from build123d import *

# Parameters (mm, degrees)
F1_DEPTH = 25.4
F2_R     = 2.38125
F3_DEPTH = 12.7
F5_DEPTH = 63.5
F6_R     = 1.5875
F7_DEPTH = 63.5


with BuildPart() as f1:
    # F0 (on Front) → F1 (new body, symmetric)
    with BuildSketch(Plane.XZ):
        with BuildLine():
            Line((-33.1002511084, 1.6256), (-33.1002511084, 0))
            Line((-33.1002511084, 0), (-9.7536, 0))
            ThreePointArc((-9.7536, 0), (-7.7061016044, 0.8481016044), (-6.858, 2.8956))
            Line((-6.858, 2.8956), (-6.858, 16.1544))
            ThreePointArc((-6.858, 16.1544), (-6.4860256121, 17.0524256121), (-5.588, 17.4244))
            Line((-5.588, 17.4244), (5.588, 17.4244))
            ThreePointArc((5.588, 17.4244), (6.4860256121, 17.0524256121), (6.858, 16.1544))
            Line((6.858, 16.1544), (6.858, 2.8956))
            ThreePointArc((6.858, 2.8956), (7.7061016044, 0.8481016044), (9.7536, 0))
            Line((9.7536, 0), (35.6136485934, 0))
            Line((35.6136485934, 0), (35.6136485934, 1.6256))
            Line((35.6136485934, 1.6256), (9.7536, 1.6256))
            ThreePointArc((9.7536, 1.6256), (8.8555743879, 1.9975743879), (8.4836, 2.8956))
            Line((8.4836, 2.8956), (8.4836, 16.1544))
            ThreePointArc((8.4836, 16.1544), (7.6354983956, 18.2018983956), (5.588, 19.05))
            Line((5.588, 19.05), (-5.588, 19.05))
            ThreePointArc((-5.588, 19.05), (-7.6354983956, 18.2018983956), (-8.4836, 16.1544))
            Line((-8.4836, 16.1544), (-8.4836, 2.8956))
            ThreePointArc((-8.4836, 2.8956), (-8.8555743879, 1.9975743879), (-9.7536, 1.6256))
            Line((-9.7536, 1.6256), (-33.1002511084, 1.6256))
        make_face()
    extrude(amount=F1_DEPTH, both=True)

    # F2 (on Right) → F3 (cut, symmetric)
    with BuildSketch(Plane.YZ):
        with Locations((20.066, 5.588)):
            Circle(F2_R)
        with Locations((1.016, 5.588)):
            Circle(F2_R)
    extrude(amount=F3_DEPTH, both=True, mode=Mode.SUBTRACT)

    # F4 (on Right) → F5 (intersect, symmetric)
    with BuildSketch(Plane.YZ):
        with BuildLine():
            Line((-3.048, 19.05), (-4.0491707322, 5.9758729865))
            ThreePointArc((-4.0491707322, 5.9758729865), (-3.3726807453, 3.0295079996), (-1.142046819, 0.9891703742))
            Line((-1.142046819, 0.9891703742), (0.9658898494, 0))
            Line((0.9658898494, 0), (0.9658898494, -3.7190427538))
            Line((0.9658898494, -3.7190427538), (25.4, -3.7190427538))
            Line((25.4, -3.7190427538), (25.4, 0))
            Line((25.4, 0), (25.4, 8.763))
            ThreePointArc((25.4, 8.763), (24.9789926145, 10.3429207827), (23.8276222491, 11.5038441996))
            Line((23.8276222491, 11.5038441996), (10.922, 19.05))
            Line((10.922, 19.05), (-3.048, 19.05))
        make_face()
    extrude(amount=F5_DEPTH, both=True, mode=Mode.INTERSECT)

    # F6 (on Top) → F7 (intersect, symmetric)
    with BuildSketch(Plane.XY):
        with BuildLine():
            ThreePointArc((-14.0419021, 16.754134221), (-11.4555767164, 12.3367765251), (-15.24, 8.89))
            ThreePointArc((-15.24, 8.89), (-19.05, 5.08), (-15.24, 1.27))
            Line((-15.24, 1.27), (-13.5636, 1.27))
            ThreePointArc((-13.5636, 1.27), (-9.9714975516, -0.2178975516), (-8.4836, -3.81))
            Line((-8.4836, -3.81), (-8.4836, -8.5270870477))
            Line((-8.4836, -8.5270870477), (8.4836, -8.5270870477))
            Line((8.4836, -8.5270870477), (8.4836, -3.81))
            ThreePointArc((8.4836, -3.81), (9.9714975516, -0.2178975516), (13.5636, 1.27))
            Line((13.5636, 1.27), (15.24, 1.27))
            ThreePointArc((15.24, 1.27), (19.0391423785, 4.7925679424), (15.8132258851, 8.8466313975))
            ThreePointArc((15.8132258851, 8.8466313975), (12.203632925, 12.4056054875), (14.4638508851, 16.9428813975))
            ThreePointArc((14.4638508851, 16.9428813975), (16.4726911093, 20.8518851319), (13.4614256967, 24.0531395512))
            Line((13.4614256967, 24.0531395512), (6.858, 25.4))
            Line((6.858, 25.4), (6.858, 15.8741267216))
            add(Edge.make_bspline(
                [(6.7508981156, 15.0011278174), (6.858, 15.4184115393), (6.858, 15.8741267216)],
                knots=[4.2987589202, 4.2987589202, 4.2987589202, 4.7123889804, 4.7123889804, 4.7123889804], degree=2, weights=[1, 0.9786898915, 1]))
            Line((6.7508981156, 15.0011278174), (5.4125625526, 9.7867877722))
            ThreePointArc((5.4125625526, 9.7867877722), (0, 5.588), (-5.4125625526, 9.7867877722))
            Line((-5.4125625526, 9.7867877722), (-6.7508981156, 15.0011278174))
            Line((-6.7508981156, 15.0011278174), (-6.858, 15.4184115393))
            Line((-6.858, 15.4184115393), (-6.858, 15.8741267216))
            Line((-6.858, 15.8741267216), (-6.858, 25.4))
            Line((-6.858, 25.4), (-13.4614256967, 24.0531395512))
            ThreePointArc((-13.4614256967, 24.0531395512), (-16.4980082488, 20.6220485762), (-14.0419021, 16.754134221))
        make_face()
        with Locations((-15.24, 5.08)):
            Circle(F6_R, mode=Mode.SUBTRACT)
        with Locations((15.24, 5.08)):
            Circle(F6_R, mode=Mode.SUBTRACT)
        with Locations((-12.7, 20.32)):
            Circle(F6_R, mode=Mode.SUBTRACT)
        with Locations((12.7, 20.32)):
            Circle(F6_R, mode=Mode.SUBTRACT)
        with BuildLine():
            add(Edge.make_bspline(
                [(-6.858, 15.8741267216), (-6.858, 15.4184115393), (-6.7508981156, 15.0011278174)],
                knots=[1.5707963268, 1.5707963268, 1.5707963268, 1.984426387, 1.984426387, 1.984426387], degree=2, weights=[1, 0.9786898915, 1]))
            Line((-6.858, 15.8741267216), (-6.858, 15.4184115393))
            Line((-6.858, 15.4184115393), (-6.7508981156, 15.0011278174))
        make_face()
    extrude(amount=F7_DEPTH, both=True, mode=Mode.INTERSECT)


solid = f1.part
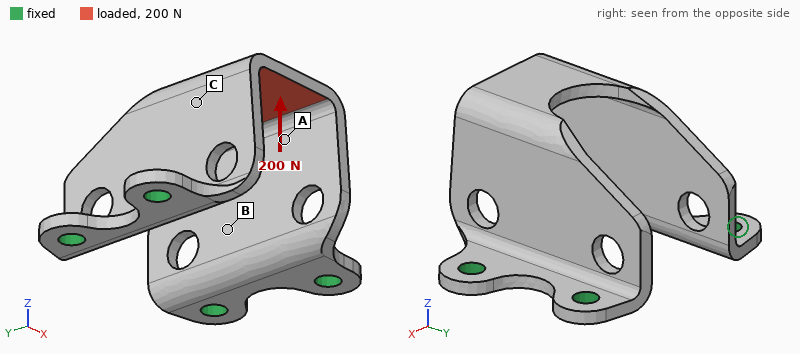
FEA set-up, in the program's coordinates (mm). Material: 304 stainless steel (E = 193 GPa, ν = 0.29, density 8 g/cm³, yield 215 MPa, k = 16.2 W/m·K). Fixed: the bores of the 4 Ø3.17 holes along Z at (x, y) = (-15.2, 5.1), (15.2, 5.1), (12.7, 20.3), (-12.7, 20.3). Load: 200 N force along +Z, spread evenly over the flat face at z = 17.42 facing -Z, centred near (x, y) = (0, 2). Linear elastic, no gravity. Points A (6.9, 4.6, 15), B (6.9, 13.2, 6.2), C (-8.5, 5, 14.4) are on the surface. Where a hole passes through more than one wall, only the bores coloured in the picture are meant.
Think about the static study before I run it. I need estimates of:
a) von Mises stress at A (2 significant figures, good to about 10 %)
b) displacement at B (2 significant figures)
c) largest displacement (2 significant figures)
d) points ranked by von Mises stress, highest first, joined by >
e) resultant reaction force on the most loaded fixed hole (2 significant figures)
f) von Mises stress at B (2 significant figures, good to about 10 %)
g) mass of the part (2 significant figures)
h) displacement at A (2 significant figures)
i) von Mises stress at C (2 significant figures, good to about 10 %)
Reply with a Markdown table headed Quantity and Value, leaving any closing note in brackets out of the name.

| Quantity | Value |
|---|---|
| von Mises stress at A | 29 MPa |
| displacement at B | 4.0 µm |
| largest displacement | 21 µm |
| points ranked by von Mises stress, highest first, joined by > | A > C > B |
| resultant reaction force on the most loaded fixed hole | 110 N |
| von Mises stress at B | 8.9 MPa |
| mass of the part | 17 g |
| displacement at A | 10 µm |
| von Mises stress at C | 16 MPa |
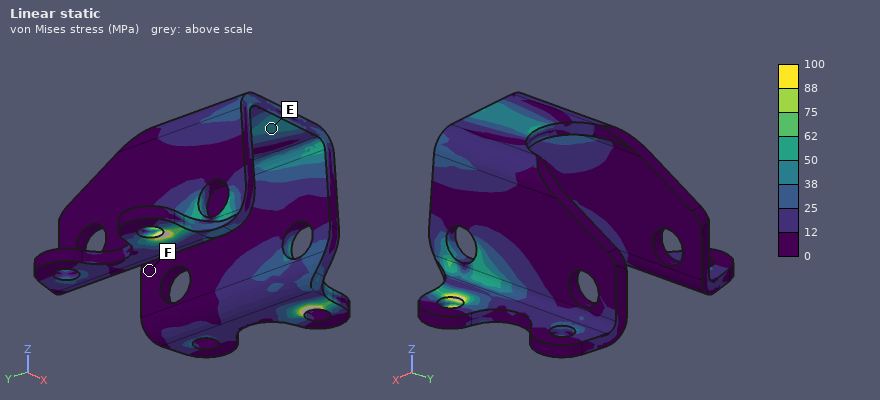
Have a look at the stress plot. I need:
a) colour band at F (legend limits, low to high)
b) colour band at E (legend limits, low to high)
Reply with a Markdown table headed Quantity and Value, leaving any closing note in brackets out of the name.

| Quantity | Value |
|---|---|
| colour band at F | 0 to 12 MPa |
| colour band at E | 38 to 50 MPa |
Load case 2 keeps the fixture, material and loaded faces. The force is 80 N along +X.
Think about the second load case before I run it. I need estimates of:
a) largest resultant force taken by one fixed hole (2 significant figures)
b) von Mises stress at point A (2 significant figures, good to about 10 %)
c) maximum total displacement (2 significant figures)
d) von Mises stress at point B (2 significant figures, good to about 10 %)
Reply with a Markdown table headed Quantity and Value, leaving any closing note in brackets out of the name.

| Quantity | Value |
|---|---|
| largest resultant force taken by one fixed hole | 45 N |
| von Mises stress at point A | 34 MPa |
| maximum total displacement | 30 µm |
| von Mises stress at point B | 17 MPa |
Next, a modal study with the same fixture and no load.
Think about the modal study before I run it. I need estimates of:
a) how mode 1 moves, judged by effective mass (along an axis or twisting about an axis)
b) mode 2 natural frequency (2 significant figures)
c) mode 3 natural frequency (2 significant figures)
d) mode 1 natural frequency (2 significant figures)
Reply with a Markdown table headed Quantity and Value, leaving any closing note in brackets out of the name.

| Quantity | Value |
|---|---|
| how mode 1 moves, judged by effective mass | along X |
| mode 2 natural frequency | 6200 Hz |
| mode 3 natural frequency | 6800 Hz |
| mode 1 natural frequency | 3800 Hz |
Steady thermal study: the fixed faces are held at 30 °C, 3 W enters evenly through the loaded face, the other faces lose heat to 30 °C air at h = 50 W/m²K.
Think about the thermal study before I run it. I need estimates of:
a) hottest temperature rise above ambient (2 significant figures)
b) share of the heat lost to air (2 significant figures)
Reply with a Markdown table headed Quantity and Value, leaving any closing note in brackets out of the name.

| Quantity | Value |
|---|---|
| hottest temperature rise above ambient | 60 K |
| share of the heat lost to air | 69 % |
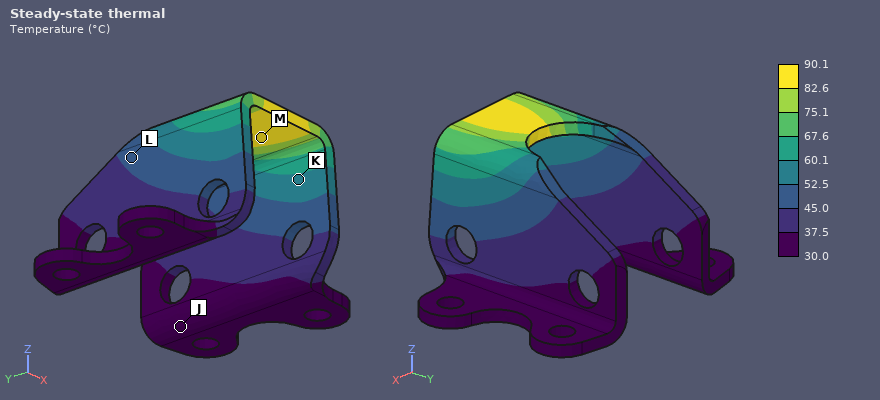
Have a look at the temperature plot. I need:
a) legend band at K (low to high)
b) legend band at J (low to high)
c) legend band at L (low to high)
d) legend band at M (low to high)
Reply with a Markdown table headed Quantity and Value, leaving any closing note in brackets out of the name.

| Quantity | Value |
|---|---|
| legend band at K | 52.5 to 60.1 °C |
| legend band at J | 30.0 to 37.5 °C |
| legend band at L | 45.0 to 52.5 °C |
| legend band at M | 82.6 to 90.1 °C |
